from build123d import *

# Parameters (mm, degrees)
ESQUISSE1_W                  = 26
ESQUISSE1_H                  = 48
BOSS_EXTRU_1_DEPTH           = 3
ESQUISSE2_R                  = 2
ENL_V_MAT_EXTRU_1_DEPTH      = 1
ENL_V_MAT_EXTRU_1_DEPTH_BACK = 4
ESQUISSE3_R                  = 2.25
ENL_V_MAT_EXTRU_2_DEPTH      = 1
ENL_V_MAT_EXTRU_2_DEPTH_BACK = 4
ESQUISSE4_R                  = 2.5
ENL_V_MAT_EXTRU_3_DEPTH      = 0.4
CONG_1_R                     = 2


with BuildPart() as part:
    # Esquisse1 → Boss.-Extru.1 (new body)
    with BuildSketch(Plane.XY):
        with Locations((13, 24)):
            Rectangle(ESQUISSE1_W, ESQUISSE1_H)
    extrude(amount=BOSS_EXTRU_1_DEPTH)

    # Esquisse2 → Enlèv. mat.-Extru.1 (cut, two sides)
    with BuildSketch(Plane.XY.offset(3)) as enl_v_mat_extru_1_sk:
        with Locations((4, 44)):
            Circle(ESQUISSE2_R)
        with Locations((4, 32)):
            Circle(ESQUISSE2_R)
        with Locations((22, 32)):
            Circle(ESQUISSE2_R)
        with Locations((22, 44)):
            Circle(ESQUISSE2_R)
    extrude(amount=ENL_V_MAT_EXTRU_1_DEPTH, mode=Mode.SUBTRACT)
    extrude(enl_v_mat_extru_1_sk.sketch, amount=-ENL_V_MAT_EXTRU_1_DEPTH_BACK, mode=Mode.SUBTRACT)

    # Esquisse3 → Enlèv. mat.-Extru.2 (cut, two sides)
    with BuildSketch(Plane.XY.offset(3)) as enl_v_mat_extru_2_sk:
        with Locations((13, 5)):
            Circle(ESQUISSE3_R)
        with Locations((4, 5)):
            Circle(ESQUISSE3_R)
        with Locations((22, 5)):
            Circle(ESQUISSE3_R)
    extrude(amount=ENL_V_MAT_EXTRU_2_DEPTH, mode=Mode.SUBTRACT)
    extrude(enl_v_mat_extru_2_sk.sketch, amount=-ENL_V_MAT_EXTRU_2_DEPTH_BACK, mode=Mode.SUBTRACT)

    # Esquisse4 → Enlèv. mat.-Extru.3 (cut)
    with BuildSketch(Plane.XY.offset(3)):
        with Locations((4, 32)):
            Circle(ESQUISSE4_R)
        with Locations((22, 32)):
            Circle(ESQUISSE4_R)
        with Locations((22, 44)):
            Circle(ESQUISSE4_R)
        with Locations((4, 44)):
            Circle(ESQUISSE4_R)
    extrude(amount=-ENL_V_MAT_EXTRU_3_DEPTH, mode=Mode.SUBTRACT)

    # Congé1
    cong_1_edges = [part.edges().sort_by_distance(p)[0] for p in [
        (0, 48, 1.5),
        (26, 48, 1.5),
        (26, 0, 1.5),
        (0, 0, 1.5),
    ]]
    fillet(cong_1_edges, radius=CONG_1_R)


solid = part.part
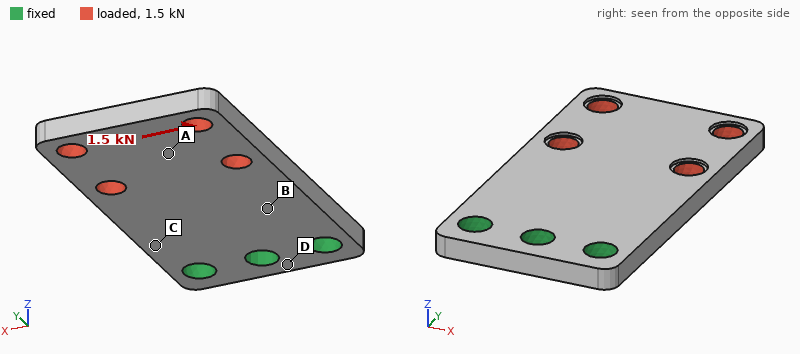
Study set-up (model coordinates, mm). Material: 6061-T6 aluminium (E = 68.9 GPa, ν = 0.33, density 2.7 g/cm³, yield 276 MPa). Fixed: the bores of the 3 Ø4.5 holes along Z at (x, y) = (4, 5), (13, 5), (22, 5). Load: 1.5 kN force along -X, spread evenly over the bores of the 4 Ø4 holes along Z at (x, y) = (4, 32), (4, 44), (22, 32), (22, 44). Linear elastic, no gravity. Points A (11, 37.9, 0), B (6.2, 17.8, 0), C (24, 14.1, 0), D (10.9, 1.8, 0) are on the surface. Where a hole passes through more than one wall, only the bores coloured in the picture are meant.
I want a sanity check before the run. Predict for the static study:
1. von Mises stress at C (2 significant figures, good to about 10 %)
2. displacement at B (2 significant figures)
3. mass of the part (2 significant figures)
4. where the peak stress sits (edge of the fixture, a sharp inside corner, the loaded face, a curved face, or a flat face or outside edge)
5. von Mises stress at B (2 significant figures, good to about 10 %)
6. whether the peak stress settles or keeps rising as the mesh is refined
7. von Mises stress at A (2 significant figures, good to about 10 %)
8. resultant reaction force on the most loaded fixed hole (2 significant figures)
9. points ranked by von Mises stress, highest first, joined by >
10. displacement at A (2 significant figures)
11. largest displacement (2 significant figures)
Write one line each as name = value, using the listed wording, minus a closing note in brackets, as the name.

von Mises stress at C = 88 MPa
displacement at B = 0.022 mm
mass of the part = 9.3 g
where the peak stress sits = edge of the fixture
von Mises stress at B = 63 MPa
whether the peak stress settles or keeps rising as the mesh is refined = keeps rising
von Mises stress at A = 28 MPa
resultant reaction force on the most loaded fixed hole = 2.5 kN
points ranked by von Mises stress, highest first, joined by > = C > B > A > D
displacement at A = 0.083 mm
largest displacement = 0.12 mm
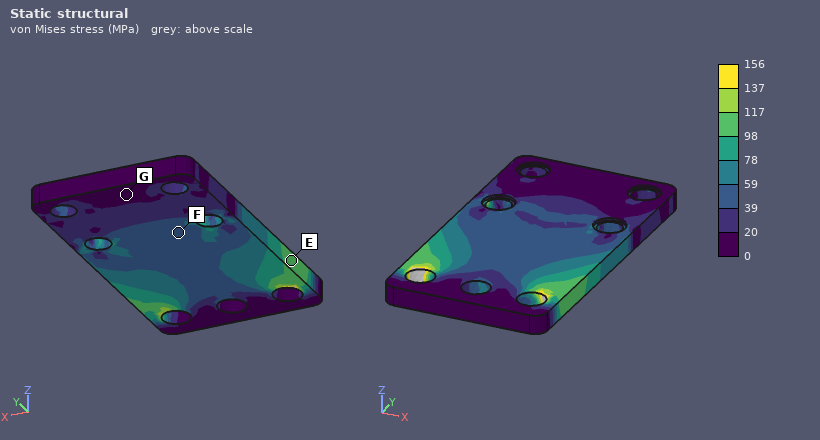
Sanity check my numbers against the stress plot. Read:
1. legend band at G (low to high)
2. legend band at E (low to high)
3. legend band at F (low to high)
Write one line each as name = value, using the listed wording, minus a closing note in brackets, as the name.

legend band at G = 0 to 20 MPa
legend band at E = 98 to 117 MPa
legend band at F = 39 to 59 MPa
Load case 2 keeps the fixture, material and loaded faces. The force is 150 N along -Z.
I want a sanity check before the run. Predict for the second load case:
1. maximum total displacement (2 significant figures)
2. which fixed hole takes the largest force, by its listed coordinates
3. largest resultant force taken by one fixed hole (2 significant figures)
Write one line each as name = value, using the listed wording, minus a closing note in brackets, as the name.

maximum total displacement = 0.56 mm
which fixed hole takes the largest force, by its listed coordinates = (13, 5)
largest resultant force taken by one fixed hole = 110 N
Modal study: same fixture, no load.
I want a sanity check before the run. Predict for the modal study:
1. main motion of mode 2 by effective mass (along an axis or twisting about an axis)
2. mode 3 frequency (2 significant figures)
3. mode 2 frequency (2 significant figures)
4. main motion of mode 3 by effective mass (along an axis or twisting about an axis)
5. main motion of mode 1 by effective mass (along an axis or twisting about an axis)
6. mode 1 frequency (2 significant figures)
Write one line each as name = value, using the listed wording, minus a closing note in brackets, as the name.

main motion of mode 2 by effective mass = twisting about Y
mode 3 frequency = 8700 Hz
mode 2 frequency = 5100 Hz
main motion of mode 3 by effective mass = along Z
main motion of mode 1 by effective mass = along Z
mode 1 frequency = 1500 Hz
